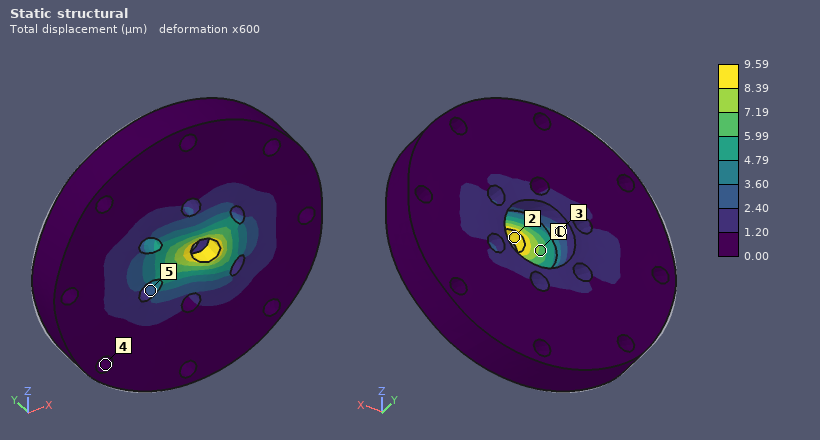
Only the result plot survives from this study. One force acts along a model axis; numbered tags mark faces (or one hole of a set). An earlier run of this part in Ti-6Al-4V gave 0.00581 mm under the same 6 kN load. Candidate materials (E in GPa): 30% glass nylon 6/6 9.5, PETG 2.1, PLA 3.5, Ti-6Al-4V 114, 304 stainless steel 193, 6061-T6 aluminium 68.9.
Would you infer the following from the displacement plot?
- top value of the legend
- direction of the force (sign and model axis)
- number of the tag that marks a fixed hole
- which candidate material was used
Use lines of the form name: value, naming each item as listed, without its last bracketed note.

top value of the legend: 9.59 µm
direction of the force: +X
number of the tag that marks a fixed hole: 4
which candidate material was used: 6061-T6 aluminium
